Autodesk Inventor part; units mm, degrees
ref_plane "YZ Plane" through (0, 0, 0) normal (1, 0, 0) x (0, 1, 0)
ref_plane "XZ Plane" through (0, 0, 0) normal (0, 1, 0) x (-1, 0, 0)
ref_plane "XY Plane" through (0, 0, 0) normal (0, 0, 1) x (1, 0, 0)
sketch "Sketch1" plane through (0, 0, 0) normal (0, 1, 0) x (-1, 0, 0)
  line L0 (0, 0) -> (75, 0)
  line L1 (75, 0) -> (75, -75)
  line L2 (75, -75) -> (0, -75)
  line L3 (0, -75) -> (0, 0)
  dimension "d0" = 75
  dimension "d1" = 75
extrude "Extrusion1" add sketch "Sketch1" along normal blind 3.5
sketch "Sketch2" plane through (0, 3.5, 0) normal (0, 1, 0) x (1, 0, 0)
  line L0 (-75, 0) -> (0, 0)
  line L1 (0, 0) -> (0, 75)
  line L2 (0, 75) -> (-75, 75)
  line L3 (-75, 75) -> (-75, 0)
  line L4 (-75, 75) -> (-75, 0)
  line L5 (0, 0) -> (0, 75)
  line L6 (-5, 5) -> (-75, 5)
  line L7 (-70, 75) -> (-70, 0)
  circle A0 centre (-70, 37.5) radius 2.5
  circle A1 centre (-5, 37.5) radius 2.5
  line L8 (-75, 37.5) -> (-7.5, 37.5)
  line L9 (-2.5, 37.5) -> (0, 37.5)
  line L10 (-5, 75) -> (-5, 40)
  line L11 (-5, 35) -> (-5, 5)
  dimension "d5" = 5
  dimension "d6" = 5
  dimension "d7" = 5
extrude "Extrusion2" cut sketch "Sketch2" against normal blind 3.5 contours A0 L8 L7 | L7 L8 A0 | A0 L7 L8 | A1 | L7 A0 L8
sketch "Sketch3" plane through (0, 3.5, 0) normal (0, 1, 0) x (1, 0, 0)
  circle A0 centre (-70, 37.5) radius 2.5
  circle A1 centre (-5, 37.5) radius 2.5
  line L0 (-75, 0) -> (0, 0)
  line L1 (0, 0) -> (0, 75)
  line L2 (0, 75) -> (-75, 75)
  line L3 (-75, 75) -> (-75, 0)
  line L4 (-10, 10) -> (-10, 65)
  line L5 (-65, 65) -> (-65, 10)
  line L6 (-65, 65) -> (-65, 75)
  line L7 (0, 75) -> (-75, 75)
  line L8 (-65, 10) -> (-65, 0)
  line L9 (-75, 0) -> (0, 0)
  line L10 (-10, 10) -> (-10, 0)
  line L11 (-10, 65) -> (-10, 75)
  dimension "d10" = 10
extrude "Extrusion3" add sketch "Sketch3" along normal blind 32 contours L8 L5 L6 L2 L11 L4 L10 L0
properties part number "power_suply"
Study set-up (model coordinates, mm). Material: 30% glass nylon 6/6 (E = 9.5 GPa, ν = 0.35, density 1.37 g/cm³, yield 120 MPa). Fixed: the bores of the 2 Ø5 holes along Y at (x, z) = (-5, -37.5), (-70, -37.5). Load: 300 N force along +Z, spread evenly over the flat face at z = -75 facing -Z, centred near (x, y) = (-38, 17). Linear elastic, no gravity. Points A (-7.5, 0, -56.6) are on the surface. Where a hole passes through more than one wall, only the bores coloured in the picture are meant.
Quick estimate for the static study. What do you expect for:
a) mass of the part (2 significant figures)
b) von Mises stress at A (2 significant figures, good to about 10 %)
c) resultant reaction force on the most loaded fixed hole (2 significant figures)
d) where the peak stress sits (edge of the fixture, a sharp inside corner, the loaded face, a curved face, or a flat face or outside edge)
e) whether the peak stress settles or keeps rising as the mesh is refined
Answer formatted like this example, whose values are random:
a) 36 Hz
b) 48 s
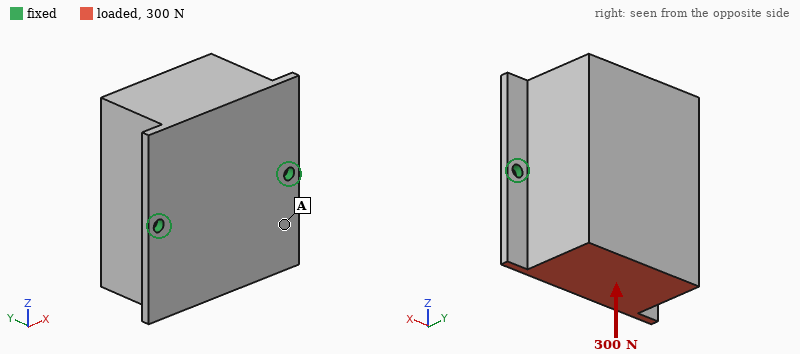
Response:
a) 210 g
b) 4.7 MPa
c) 150 N
d) edge of the fixture
e) keeps rising
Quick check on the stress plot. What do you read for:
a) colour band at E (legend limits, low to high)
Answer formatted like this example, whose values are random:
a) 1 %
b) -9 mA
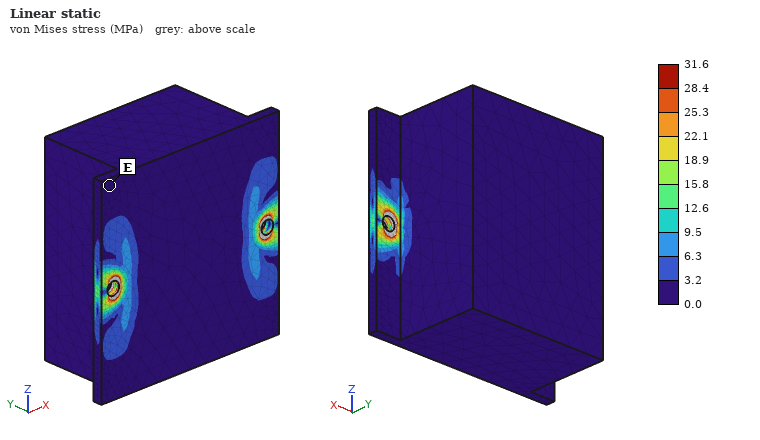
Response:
a) 0.0 to 3.2 MPa
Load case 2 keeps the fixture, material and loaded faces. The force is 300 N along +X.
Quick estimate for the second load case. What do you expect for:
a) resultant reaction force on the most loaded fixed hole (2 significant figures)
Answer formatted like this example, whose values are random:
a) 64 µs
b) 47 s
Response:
a) 240 N
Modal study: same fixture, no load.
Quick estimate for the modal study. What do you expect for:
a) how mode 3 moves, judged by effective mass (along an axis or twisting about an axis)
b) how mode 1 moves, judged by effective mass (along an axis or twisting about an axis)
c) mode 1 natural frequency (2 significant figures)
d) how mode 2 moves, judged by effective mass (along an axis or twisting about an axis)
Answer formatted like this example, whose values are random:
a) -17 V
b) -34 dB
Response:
a) along X
b) along Z
c) 310 Hz
d) along Y
